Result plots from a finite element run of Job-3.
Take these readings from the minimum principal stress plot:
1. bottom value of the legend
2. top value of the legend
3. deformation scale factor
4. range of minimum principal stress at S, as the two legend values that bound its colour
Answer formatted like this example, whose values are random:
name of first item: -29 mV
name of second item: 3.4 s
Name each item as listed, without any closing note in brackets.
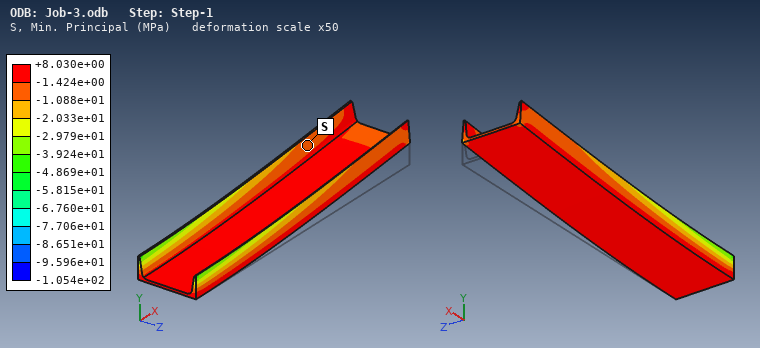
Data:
bottom value of the legend: -1.054e+02 MPa
top value of the legend: +8.030e+00 MPa
deformation scale factor: 50
range of minimum principal stress at S, as the two legend values that bound its colour: -1.088e+01 to -1.424e+00 MPa
